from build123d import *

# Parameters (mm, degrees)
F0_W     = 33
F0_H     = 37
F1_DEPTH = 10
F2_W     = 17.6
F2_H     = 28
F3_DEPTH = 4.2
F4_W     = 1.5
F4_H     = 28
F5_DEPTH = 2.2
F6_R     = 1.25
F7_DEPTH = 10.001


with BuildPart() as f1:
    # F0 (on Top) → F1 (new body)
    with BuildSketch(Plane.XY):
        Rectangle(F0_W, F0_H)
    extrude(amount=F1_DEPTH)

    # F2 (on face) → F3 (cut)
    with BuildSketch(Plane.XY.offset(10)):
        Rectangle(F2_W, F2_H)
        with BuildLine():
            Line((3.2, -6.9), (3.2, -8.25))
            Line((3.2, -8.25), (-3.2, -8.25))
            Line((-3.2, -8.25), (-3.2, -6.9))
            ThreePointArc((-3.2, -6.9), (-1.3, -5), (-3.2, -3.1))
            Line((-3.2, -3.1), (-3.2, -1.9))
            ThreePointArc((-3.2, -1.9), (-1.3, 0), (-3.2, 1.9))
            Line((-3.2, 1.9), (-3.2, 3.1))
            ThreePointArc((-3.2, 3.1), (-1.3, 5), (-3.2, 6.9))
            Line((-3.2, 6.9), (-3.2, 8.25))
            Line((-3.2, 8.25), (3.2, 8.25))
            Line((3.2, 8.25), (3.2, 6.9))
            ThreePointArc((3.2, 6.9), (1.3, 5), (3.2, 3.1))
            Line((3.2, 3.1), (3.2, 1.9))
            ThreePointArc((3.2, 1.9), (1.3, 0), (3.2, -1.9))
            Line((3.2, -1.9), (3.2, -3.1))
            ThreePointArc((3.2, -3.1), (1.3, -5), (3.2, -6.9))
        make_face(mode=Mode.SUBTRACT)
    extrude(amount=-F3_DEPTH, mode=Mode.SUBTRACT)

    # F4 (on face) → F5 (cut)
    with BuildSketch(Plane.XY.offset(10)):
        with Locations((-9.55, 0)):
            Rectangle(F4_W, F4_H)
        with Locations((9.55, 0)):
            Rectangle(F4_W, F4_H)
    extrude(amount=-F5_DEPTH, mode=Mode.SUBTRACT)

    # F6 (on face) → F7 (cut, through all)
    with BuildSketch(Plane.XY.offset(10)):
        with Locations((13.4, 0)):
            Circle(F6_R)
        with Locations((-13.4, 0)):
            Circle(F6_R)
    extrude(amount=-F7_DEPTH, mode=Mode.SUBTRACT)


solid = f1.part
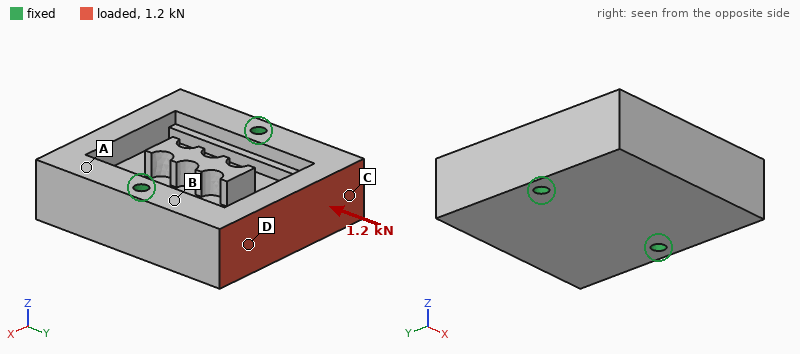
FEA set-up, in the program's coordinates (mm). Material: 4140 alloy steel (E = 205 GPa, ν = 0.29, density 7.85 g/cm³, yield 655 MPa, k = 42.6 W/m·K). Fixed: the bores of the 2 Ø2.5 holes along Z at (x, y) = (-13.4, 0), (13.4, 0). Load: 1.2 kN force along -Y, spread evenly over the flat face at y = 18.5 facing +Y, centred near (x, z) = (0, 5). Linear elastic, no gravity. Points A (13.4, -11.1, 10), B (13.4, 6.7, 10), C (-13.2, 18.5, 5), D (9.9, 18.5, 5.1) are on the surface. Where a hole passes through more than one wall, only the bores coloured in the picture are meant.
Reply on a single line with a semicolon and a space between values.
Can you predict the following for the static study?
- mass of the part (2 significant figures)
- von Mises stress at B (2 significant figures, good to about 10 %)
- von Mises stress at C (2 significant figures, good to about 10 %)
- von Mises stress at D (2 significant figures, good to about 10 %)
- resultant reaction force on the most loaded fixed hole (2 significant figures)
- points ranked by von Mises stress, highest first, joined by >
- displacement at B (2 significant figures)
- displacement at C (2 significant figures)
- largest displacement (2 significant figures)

80 g; 8.5 MPa; 4.9 MPa; 6.5 MPa; 600 N; B > D > C > A; 0.30 µm; 0.62 µm; 1.6 µm
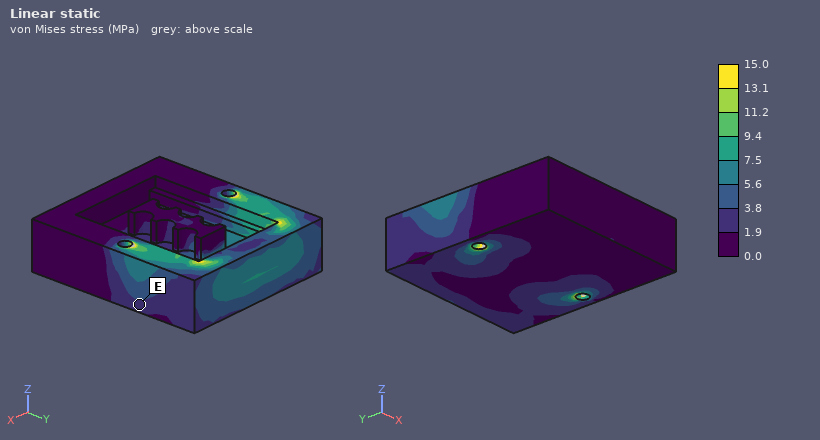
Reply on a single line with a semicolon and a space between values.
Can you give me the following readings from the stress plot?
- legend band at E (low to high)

1.9 to 3.8 MPa
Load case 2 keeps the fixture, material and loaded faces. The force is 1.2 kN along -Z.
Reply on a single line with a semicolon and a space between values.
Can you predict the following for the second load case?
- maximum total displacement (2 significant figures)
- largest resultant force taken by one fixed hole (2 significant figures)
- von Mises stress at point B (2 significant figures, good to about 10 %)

13 µm; 610 N; 50 MPa
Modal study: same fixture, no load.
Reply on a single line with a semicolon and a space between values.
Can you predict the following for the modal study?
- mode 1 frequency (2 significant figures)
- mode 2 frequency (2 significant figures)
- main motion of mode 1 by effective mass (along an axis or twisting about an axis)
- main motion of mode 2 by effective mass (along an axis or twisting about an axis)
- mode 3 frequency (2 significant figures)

13 kHz; 16 kHz; twisting about X; along Z; 22 kHz
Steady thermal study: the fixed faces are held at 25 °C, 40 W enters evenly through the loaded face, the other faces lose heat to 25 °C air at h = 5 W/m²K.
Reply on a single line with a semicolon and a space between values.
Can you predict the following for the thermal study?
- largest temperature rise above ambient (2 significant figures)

82 K
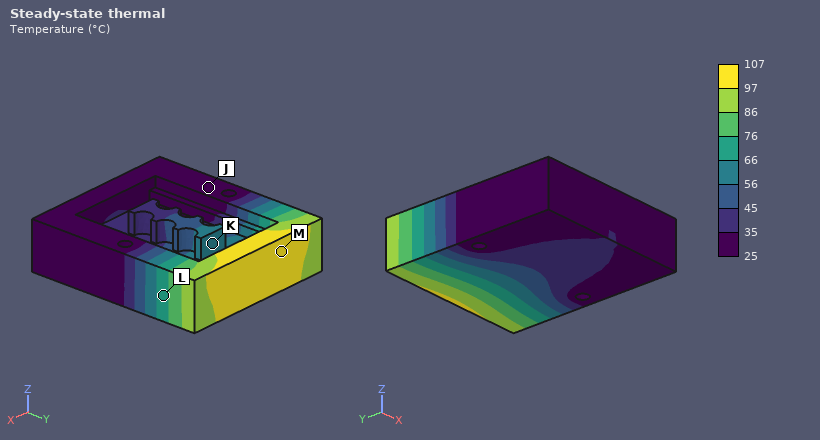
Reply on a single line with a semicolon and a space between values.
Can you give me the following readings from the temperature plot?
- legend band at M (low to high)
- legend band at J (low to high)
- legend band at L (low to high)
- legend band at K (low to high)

97 to 107 °C; 25 to 35 °C; 66 to 76 °C; 56 to 66 °C
